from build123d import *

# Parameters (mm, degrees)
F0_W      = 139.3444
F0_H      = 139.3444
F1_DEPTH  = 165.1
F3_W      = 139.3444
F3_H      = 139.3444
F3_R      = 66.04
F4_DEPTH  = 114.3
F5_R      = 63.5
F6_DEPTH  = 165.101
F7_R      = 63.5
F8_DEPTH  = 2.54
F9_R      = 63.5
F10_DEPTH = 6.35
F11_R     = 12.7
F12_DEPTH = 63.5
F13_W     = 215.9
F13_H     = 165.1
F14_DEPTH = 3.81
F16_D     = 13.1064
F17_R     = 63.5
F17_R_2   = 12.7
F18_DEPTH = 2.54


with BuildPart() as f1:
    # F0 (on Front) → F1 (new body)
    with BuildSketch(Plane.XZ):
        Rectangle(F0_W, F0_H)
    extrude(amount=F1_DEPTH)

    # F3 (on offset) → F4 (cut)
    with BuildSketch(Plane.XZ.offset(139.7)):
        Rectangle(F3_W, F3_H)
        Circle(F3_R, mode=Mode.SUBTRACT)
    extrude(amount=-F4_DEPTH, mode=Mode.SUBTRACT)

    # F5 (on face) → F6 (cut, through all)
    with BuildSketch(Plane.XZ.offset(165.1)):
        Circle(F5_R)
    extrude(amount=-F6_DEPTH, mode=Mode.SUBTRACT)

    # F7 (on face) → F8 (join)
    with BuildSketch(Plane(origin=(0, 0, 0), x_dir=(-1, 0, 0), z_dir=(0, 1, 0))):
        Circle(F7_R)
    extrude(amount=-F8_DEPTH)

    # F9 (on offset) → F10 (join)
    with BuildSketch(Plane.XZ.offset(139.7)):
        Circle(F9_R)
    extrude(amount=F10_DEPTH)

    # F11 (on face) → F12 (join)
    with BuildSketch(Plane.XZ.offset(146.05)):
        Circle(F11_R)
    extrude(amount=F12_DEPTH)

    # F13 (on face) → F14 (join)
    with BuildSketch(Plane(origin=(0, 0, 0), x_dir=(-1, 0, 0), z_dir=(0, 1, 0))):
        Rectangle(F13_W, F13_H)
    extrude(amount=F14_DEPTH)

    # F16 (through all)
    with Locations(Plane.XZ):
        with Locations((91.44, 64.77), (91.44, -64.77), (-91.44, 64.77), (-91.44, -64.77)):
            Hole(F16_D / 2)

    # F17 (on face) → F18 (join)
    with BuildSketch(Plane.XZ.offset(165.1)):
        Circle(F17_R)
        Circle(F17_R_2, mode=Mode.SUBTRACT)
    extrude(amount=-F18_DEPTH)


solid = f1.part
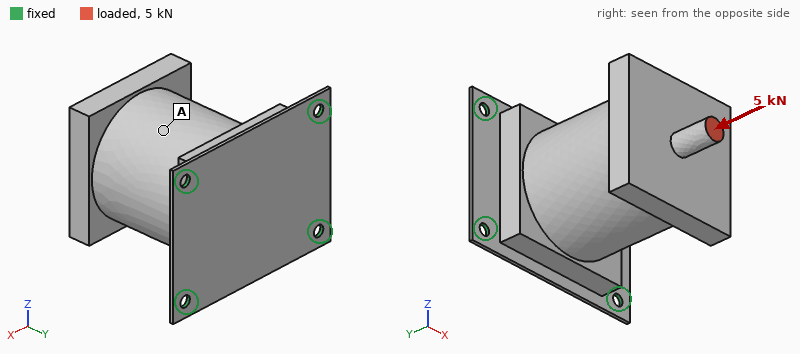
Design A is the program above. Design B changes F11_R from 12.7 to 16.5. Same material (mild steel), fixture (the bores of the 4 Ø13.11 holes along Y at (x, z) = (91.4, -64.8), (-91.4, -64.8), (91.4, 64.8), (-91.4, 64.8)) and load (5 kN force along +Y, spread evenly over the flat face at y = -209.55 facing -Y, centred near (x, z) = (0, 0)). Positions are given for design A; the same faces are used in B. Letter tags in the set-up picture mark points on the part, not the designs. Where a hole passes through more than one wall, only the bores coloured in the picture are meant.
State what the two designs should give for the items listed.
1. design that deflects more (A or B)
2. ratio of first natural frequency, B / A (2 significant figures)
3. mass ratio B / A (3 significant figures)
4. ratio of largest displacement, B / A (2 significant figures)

A
0.96
1.03
0.87
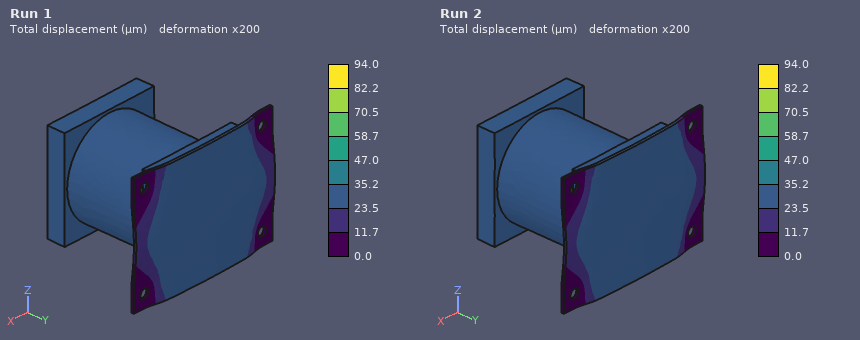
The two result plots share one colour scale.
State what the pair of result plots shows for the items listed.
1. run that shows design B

Run 2
